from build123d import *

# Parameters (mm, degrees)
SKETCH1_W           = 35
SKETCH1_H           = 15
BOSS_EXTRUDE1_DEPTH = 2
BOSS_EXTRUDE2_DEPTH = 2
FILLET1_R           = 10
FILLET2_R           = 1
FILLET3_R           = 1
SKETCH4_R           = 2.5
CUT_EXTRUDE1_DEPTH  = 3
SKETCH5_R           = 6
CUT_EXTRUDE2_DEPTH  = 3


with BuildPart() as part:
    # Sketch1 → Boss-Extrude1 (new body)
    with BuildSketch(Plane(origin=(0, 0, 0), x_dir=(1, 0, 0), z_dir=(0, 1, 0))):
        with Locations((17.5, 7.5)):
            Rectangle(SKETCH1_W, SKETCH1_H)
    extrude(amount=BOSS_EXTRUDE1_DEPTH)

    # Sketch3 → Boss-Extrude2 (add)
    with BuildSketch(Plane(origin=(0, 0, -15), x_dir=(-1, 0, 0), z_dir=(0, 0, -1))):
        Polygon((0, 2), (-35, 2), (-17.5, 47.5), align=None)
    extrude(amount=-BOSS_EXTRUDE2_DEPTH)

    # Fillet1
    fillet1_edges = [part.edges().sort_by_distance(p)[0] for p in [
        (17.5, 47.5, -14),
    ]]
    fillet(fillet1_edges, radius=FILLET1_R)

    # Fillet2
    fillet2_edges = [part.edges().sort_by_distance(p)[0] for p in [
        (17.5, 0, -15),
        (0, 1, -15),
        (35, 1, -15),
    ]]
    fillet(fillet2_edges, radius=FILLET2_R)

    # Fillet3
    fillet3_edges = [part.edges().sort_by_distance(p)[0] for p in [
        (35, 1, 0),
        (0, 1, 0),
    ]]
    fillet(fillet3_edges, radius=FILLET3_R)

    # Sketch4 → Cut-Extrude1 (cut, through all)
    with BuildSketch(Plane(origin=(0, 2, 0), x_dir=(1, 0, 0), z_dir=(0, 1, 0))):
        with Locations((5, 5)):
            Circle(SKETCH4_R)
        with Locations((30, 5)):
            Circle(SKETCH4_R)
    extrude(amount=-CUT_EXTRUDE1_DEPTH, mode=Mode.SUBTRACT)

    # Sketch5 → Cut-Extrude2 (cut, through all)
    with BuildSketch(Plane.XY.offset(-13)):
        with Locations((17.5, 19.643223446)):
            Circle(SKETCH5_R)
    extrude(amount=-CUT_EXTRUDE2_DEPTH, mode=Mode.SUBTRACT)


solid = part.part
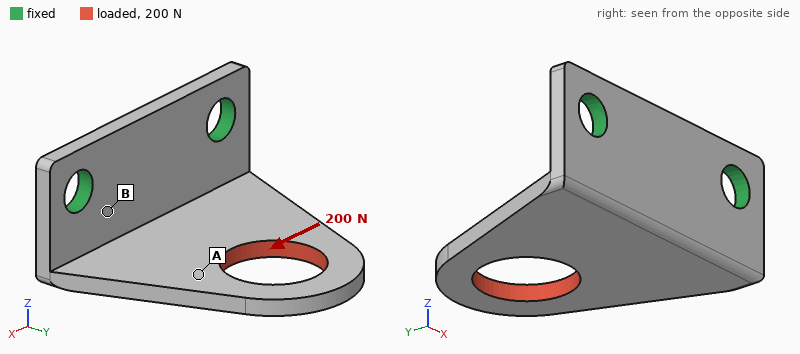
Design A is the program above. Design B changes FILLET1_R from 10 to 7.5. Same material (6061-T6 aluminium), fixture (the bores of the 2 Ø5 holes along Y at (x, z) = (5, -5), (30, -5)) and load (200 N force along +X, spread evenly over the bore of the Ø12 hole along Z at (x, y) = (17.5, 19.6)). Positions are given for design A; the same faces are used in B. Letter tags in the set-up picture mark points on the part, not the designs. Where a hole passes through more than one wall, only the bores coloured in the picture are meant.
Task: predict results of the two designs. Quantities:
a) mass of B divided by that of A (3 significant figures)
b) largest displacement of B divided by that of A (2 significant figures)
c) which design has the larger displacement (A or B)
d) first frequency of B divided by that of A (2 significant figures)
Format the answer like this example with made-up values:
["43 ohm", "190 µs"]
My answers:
["1.06", "1.1", "B", "0.75"]
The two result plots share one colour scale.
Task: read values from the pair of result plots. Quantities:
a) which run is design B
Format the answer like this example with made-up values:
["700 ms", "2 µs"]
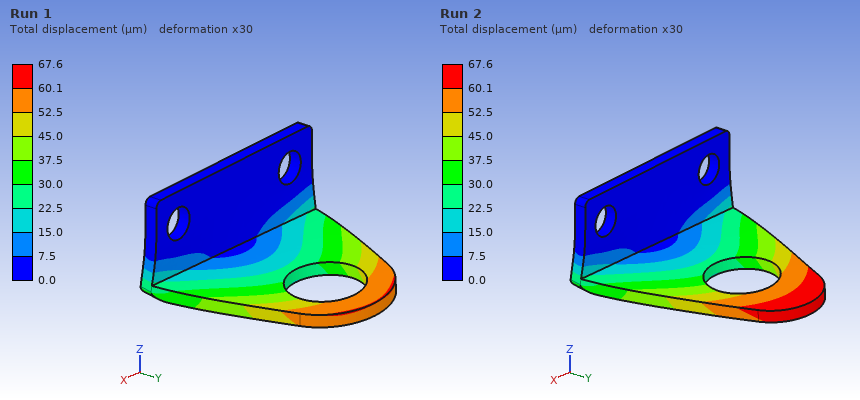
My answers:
["Run 2"]
